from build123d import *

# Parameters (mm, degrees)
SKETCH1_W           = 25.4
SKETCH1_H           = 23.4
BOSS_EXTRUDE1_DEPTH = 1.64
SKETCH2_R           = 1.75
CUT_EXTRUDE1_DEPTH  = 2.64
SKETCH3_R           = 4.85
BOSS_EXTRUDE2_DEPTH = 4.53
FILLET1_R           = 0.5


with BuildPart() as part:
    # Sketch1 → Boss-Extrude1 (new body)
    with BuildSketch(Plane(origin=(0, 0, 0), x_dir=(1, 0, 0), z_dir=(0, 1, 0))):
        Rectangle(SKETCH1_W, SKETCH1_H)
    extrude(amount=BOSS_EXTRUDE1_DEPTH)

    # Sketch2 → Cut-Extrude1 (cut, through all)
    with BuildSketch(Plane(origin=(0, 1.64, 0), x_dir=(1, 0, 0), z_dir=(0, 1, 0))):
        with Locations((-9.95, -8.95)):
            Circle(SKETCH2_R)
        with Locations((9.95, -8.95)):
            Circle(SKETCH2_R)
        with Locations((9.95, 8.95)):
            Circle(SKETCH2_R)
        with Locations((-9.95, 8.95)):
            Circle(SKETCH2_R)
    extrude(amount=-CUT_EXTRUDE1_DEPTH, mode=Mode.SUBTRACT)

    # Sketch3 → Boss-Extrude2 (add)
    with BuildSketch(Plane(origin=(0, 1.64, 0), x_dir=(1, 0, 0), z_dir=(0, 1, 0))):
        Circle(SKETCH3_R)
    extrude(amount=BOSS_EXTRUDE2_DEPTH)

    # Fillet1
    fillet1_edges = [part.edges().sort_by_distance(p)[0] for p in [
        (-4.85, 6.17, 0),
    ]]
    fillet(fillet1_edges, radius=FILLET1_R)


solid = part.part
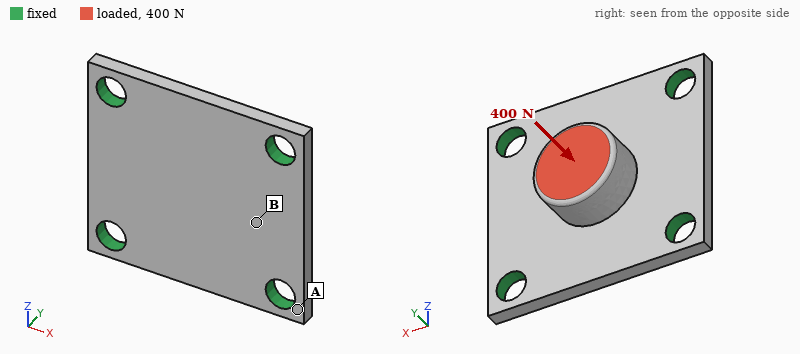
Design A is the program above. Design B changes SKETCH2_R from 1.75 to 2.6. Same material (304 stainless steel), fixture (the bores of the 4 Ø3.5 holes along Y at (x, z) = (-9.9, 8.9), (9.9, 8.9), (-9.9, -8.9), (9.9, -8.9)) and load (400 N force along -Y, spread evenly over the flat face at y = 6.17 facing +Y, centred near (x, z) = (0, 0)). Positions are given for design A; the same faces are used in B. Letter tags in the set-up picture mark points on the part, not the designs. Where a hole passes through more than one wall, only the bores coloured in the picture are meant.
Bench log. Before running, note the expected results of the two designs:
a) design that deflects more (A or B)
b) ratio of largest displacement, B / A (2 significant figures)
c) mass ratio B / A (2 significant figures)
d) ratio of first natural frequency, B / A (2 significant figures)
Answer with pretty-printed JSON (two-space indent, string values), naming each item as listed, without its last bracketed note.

{
  "design that deflects more": "A",
  "ratio of largest displacement, B / A": "0.73",
  "mass ratio B / A": "0.94",
  "ratio of first natural frequency, B / A": "1.2"
}
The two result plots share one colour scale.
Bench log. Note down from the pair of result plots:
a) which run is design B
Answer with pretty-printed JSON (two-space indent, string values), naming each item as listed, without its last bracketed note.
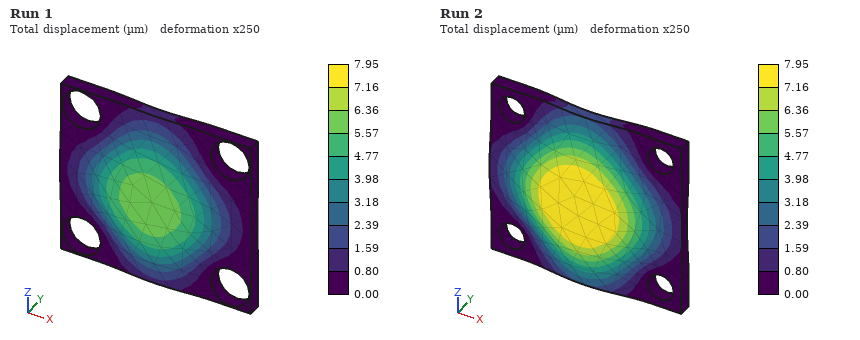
{
  "which run is design B": "Run 1"
}
